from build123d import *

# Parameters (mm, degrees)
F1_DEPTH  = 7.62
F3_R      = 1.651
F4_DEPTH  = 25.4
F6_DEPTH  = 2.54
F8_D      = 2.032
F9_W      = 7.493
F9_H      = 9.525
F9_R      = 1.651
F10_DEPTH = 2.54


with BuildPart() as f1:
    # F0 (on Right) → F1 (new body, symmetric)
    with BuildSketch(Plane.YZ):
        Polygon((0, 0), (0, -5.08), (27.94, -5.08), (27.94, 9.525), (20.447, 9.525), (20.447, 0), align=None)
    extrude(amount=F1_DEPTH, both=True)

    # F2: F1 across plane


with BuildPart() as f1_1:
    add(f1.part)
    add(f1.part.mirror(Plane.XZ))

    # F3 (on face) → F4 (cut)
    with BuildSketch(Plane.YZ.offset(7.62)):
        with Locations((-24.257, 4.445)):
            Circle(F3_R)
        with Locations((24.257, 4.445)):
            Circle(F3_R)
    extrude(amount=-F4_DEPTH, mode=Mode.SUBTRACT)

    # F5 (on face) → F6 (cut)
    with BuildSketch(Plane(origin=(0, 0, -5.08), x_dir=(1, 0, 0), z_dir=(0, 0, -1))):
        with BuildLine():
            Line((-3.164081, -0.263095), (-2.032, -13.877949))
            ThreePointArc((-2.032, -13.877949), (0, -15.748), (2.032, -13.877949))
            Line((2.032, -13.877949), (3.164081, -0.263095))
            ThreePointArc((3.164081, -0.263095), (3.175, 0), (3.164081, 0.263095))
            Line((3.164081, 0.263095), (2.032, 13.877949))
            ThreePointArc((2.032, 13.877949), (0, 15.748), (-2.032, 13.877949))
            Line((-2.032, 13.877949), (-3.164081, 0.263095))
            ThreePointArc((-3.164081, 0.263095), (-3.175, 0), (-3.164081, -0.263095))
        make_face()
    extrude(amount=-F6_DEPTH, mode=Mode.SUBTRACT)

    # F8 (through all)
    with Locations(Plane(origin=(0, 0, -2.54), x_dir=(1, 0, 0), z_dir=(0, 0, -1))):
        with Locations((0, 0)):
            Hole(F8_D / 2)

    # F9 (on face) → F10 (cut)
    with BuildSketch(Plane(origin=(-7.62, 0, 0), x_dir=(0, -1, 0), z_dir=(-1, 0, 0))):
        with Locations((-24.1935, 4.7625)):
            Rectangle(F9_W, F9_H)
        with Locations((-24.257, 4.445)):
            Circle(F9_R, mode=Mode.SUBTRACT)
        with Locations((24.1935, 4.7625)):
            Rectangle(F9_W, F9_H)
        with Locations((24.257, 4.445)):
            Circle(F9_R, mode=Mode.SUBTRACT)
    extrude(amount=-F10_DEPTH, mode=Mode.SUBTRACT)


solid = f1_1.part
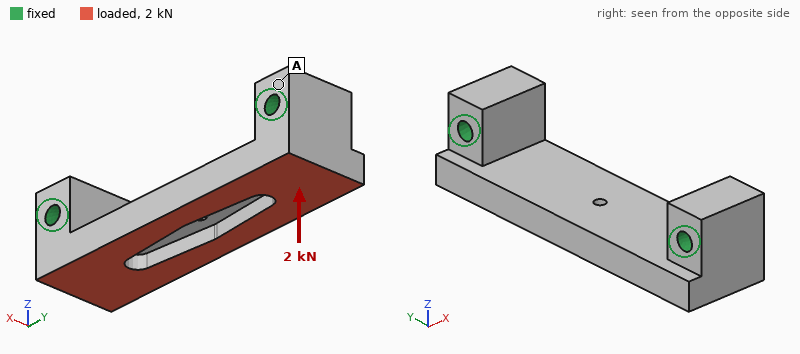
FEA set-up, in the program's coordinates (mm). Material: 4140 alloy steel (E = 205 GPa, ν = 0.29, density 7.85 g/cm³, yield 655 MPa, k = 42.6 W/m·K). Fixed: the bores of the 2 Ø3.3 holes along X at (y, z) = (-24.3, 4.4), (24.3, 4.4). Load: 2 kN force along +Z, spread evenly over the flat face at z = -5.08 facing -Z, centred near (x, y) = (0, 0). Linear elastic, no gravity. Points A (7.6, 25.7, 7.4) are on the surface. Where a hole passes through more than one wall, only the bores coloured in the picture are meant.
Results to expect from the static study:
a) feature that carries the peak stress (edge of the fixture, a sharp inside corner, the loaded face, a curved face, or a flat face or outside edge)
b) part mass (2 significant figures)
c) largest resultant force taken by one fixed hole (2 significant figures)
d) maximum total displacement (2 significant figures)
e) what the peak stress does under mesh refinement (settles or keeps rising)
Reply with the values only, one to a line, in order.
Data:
a sharp inside corner
43 g
1.1 kN
17 µm
keeps rising
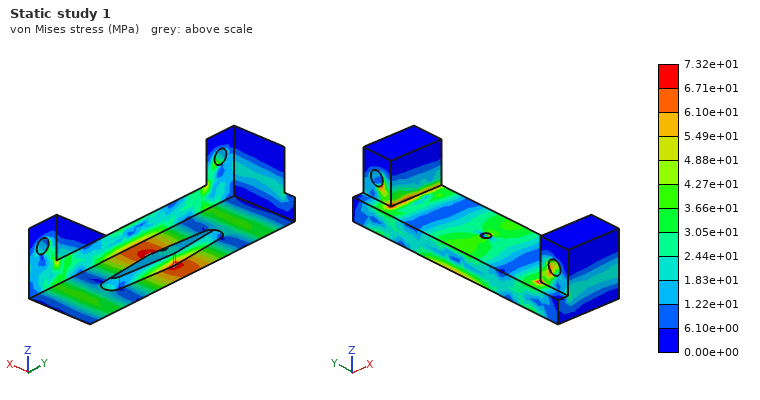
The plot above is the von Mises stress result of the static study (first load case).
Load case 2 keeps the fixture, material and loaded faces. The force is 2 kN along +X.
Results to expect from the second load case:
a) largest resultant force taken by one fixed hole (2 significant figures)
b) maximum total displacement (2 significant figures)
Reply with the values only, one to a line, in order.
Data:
1.0 kN
11 µm
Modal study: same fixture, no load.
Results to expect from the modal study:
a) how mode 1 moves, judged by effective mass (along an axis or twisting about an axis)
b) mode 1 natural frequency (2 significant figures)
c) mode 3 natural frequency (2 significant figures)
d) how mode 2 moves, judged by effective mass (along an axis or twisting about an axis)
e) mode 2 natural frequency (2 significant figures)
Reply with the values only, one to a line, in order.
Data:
along Z
11 kHz
19 kHz
along X
18 kHz
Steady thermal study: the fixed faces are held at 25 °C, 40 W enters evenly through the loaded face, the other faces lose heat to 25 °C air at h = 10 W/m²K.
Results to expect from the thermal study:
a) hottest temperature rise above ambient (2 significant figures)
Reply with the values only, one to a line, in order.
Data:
76 K
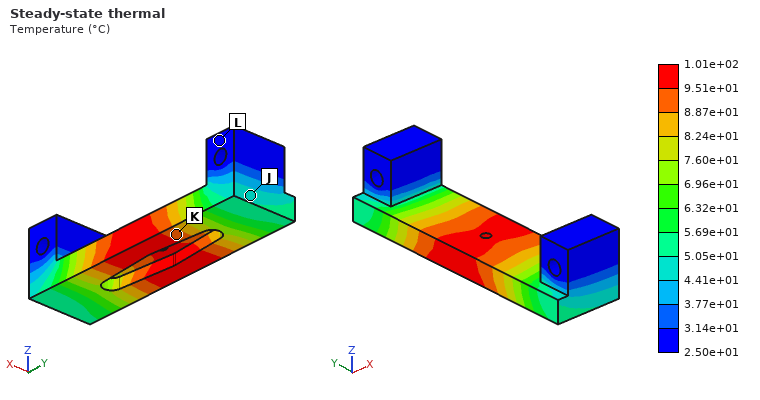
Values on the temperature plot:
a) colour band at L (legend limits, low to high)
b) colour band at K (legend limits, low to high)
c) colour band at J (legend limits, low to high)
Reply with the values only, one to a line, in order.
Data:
2.50e+01 to 3.14e+01 °C
8.87e+01 to 9.51e+01 °C
4.41e+01 to 5.05e+01 °C
